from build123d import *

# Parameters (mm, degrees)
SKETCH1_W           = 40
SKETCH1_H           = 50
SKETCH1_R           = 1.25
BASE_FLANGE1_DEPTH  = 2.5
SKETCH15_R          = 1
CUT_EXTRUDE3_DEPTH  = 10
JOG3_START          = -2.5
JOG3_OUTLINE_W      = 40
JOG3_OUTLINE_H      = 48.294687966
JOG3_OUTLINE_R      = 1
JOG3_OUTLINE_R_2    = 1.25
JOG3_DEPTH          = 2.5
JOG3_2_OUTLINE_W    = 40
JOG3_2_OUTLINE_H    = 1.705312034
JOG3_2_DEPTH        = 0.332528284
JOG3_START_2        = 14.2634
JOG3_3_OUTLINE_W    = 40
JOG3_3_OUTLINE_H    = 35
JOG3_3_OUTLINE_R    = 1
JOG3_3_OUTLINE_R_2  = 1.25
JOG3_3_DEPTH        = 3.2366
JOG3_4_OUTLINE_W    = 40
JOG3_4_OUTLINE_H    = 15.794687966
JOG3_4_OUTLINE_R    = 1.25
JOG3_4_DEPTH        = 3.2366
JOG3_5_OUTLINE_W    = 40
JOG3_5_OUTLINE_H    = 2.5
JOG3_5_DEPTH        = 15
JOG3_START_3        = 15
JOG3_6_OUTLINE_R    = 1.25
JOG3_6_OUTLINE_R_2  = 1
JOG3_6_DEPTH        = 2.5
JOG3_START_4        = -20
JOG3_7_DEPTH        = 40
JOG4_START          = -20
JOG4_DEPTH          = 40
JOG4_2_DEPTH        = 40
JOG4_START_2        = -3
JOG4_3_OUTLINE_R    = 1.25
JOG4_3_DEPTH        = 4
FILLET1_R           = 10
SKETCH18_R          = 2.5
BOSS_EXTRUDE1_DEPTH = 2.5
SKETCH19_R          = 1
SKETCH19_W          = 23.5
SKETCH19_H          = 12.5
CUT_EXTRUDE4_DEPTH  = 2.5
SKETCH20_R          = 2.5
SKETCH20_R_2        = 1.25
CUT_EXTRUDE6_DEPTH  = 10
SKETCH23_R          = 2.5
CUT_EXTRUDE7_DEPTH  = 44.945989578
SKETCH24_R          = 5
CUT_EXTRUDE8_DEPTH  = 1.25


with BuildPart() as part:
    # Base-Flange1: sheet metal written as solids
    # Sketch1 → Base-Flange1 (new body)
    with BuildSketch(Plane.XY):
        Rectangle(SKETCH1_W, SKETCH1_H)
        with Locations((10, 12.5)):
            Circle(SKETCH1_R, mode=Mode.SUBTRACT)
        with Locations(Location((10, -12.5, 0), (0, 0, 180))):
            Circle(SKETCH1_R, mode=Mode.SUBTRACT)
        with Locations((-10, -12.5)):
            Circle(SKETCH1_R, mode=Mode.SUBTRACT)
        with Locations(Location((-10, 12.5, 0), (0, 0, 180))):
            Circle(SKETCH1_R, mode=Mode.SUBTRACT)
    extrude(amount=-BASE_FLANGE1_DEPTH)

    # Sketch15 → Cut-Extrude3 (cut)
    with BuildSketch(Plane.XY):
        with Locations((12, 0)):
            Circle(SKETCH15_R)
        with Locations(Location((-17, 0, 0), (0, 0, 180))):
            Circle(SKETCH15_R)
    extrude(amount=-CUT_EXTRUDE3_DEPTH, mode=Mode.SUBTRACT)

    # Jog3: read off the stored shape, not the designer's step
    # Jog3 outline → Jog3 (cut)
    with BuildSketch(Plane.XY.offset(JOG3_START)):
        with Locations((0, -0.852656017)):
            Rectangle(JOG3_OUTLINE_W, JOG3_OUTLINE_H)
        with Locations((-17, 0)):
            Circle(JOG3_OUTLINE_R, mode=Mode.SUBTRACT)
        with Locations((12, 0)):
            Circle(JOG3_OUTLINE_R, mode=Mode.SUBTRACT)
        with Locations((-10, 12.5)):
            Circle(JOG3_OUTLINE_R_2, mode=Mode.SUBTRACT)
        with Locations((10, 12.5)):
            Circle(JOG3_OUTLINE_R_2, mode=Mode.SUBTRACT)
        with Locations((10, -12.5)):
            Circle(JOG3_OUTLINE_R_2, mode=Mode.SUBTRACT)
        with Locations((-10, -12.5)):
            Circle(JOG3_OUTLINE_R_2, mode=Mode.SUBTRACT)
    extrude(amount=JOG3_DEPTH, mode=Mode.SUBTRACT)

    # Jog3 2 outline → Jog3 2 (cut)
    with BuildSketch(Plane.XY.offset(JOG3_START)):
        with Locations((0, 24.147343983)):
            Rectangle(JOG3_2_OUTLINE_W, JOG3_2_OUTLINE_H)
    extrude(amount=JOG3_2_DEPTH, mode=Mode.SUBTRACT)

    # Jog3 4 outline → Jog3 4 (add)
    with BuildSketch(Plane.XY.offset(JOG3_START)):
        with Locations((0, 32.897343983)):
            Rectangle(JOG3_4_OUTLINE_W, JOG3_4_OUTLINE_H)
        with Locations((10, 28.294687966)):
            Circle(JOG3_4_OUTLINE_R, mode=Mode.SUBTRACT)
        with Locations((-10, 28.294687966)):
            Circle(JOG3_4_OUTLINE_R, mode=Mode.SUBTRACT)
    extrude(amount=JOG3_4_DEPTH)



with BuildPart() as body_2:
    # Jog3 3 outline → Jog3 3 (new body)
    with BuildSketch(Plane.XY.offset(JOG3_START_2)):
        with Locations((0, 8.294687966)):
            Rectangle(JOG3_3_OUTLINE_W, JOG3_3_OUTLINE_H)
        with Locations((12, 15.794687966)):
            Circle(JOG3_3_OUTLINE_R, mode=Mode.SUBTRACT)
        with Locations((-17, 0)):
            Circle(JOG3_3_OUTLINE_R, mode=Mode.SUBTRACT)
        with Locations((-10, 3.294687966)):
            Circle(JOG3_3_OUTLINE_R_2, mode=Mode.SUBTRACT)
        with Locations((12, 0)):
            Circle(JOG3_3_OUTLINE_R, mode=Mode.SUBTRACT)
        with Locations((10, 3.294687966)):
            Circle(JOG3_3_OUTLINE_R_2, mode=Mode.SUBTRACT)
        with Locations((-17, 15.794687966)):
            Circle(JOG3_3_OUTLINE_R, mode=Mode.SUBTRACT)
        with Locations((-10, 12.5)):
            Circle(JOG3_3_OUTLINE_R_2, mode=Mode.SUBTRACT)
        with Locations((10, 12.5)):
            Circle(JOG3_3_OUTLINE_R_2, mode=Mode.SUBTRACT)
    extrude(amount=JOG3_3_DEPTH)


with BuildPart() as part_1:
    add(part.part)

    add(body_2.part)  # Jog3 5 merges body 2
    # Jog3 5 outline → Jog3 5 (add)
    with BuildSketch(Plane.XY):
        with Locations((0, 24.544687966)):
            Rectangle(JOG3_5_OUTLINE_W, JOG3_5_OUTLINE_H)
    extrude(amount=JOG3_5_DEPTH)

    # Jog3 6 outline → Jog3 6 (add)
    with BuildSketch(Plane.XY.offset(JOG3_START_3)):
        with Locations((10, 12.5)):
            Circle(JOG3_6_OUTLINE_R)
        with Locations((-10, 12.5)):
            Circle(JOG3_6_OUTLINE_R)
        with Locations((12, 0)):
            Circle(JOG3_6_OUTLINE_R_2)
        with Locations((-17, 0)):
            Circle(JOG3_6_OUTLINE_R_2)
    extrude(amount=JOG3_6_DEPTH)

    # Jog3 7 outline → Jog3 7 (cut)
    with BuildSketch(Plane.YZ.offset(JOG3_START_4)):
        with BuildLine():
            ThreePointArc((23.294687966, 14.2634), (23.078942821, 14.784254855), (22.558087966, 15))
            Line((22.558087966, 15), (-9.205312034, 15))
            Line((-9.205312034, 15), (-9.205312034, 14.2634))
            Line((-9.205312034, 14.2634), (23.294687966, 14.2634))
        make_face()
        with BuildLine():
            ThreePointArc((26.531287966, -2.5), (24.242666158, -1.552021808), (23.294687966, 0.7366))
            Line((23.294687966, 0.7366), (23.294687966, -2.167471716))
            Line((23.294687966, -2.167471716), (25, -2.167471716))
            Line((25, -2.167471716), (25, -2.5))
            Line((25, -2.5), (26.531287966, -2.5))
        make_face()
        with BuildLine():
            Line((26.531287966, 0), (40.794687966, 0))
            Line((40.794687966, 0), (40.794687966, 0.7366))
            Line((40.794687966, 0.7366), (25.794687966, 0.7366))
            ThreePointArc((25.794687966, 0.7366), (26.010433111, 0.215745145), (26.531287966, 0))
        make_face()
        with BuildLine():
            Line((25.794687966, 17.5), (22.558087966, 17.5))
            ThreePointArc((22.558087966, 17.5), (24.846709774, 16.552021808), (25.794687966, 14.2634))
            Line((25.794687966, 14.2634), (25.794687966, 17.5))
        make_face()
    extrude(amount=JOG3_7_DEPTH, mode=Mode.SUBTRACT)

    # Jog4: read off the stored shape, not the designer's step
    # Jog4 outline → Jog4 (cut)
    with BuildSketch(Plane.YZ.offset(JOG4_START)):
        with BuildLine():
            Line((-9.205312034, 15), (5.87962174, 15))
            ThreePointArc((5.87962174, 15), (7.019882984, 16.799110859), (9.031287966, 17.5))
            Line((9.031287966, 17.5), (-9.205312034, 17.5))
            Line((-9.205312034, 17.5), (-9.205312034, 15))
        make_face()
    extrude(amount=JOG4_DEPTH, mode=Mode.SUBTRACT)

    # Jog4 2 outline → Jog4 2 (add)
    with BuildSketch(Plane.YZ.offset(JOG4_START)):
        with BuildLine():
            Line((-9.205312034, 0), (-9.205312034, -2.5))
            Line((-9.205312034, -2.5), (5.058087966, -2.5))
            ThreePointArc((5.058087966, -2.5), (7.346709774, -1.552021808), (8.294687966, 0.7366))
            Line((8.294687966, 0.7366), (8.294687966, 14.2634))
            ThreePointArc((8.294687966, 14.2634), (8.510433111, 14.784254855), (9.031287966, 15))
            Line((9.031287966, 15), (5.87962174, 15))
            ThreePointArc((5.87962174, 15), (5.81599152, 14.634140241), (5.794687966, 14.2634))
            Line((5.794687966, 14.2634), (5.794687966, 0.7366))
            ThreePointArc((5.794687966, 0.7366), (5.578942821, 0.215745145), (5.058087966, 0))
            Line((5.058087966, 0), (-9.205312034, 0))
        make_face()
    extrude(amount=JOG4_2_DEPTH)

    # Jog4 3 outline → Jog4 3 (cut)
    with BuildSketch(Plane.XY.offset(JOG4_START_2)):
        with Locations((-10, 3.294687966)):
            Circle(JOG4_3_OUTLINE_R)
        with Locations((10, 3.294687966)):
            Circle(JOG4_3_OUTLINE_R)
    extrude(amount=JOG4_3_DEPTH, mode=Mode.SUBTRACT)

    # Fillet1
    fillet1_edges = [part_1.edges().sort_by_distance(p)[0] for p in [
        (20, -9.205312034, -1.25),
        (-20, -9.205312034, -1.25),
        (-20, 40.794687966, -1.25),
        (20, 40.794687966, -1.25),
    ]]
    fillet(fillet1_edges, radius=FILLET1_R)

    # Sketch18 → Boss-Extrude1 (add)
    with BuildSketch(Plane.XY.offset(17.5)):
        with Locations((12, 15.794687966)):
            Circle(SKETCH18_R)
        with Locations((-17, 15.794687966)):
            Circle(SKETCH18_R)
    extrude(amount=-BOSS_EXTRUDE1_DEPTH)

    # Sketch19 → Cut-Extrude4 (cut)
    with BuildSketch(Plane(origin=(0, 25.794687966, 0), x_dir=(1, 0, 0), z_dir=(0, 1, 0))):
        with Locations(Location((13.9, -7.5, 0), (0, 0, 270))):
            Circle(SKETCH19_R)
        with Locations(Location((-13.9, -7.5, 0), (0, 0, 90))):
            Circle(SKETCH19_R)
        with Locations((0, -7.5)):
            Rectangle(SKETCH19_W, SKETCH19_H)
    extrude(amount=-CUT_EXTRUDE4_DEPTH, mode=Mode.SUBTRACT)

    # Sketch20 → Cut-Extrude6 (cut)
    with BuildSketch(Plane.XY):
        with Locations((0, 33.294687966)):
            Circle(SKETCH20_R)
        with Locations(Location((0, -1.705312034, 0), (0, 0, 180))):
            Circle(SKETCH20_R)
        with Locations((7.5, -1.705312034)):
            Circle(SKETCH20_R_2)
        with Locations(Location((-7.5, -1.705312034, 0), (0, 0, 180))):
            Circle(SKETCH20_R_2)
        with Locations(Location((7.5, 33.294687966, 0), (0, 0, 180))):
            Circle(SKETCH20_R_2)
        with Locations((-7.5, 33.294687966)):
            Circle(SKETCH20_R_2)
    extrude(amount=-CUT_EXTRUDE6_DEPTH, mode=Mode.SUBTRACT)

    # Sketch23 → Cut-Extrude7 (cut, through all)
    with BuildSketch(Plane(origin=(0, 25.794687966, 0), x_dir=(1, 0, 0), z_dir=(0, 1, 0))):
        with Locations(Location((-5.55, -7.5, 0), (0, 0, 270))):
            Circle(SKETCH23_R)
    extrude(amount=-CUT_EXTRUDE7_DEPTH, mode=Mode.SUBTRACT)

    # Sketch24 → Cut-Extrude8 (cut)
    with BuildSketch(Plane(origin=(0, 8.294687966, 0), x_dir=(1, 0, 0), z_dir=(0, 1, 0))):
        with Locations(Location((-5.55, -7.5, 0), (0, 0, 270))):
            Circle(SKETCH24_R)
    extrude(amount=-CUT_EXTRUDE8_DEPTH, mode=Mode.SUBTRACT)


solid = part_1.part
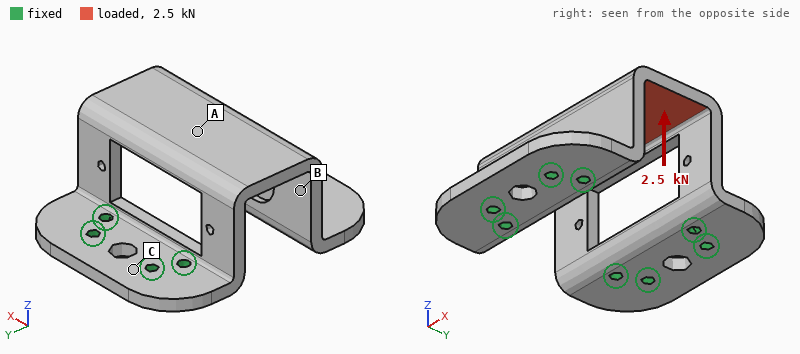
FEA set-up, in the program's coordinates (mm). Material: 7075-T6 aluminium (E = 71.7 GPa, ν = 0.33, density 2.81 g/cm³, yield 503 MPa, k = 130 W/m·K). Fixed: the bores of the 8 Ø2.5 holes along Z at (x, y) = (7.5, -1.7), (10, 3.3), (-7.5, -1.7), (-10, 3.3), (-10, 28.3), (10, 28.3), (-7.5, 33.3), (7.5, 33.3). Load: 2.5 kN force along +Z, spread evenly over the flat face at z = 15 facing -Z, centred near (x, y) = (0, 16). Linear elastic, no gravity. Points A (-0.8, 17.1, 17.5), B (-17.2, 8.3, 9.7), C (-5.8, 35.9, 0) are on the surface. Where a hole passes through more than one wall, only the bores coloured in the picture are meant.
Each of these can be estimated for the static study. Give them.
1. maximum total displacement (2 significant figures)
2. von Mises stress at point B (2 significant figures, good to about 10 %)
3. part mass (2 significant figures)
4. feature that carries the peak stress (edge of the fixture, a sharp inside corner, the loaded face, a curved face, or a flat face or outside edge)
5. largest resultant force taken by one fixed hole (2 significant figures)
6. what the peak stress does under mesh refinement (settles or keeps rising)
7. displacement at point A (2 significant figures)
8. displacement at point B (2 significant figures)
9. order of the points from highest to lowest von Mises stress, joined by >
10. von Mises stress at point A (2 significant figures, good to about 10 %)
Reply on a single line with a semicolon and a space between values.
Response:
84 µm; 41 MPa; 19 g; edge of the fixture; 690 N; keeps rising; 82 µm; 18 µm; A > B > C; 92 MPa
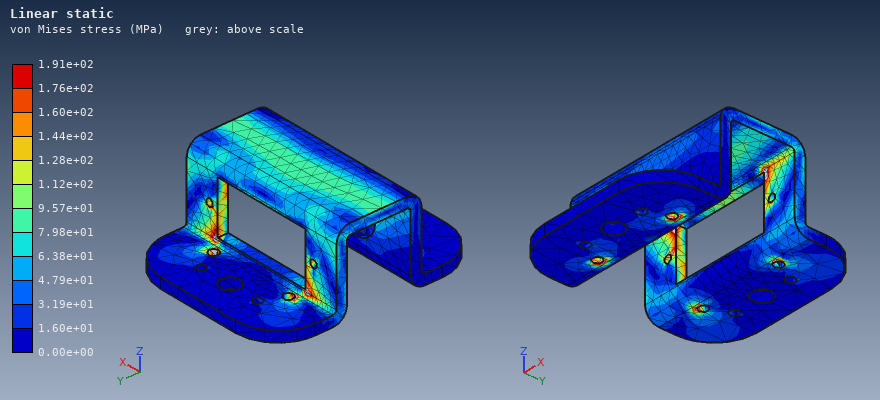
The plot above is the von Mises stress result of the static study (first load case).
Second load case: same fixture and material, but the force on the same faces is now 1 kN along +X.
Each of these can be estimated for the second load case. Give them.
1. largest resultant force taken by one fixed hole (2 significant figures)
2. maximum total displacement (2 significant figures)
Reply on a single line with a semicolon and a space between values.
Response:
780 N; 94 µm
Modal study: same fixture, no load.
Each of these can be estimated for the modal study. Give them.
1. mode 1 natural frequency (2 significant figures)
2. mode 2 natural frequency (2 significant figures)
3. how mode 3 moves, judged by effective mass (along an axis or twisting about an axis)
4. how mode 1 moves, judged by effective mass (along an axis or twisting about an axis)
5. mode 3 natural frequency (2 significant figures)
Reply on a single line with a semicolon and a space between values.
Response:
4900 Hz; 6000 Hz; along X; along Y; 10 kHz
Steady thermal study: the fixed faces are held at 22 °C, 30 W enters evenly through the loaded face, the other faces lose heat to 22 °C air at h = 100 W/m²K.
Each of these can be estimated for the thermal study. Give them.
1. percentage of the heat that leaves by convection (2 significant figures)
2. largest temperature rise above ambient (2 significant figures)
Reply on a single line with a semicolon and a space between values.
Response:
26 %; 39 K
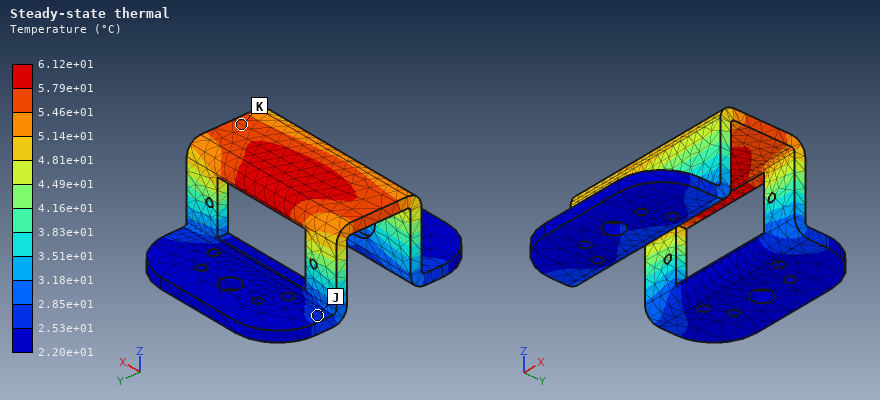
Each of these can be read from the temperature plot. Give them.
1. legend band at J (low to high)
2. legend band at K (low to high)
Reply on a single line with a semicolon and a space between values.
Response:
2.53e+01 to 2.85e+01 °C; 5.46e+01 to 5.79e+01 °C
